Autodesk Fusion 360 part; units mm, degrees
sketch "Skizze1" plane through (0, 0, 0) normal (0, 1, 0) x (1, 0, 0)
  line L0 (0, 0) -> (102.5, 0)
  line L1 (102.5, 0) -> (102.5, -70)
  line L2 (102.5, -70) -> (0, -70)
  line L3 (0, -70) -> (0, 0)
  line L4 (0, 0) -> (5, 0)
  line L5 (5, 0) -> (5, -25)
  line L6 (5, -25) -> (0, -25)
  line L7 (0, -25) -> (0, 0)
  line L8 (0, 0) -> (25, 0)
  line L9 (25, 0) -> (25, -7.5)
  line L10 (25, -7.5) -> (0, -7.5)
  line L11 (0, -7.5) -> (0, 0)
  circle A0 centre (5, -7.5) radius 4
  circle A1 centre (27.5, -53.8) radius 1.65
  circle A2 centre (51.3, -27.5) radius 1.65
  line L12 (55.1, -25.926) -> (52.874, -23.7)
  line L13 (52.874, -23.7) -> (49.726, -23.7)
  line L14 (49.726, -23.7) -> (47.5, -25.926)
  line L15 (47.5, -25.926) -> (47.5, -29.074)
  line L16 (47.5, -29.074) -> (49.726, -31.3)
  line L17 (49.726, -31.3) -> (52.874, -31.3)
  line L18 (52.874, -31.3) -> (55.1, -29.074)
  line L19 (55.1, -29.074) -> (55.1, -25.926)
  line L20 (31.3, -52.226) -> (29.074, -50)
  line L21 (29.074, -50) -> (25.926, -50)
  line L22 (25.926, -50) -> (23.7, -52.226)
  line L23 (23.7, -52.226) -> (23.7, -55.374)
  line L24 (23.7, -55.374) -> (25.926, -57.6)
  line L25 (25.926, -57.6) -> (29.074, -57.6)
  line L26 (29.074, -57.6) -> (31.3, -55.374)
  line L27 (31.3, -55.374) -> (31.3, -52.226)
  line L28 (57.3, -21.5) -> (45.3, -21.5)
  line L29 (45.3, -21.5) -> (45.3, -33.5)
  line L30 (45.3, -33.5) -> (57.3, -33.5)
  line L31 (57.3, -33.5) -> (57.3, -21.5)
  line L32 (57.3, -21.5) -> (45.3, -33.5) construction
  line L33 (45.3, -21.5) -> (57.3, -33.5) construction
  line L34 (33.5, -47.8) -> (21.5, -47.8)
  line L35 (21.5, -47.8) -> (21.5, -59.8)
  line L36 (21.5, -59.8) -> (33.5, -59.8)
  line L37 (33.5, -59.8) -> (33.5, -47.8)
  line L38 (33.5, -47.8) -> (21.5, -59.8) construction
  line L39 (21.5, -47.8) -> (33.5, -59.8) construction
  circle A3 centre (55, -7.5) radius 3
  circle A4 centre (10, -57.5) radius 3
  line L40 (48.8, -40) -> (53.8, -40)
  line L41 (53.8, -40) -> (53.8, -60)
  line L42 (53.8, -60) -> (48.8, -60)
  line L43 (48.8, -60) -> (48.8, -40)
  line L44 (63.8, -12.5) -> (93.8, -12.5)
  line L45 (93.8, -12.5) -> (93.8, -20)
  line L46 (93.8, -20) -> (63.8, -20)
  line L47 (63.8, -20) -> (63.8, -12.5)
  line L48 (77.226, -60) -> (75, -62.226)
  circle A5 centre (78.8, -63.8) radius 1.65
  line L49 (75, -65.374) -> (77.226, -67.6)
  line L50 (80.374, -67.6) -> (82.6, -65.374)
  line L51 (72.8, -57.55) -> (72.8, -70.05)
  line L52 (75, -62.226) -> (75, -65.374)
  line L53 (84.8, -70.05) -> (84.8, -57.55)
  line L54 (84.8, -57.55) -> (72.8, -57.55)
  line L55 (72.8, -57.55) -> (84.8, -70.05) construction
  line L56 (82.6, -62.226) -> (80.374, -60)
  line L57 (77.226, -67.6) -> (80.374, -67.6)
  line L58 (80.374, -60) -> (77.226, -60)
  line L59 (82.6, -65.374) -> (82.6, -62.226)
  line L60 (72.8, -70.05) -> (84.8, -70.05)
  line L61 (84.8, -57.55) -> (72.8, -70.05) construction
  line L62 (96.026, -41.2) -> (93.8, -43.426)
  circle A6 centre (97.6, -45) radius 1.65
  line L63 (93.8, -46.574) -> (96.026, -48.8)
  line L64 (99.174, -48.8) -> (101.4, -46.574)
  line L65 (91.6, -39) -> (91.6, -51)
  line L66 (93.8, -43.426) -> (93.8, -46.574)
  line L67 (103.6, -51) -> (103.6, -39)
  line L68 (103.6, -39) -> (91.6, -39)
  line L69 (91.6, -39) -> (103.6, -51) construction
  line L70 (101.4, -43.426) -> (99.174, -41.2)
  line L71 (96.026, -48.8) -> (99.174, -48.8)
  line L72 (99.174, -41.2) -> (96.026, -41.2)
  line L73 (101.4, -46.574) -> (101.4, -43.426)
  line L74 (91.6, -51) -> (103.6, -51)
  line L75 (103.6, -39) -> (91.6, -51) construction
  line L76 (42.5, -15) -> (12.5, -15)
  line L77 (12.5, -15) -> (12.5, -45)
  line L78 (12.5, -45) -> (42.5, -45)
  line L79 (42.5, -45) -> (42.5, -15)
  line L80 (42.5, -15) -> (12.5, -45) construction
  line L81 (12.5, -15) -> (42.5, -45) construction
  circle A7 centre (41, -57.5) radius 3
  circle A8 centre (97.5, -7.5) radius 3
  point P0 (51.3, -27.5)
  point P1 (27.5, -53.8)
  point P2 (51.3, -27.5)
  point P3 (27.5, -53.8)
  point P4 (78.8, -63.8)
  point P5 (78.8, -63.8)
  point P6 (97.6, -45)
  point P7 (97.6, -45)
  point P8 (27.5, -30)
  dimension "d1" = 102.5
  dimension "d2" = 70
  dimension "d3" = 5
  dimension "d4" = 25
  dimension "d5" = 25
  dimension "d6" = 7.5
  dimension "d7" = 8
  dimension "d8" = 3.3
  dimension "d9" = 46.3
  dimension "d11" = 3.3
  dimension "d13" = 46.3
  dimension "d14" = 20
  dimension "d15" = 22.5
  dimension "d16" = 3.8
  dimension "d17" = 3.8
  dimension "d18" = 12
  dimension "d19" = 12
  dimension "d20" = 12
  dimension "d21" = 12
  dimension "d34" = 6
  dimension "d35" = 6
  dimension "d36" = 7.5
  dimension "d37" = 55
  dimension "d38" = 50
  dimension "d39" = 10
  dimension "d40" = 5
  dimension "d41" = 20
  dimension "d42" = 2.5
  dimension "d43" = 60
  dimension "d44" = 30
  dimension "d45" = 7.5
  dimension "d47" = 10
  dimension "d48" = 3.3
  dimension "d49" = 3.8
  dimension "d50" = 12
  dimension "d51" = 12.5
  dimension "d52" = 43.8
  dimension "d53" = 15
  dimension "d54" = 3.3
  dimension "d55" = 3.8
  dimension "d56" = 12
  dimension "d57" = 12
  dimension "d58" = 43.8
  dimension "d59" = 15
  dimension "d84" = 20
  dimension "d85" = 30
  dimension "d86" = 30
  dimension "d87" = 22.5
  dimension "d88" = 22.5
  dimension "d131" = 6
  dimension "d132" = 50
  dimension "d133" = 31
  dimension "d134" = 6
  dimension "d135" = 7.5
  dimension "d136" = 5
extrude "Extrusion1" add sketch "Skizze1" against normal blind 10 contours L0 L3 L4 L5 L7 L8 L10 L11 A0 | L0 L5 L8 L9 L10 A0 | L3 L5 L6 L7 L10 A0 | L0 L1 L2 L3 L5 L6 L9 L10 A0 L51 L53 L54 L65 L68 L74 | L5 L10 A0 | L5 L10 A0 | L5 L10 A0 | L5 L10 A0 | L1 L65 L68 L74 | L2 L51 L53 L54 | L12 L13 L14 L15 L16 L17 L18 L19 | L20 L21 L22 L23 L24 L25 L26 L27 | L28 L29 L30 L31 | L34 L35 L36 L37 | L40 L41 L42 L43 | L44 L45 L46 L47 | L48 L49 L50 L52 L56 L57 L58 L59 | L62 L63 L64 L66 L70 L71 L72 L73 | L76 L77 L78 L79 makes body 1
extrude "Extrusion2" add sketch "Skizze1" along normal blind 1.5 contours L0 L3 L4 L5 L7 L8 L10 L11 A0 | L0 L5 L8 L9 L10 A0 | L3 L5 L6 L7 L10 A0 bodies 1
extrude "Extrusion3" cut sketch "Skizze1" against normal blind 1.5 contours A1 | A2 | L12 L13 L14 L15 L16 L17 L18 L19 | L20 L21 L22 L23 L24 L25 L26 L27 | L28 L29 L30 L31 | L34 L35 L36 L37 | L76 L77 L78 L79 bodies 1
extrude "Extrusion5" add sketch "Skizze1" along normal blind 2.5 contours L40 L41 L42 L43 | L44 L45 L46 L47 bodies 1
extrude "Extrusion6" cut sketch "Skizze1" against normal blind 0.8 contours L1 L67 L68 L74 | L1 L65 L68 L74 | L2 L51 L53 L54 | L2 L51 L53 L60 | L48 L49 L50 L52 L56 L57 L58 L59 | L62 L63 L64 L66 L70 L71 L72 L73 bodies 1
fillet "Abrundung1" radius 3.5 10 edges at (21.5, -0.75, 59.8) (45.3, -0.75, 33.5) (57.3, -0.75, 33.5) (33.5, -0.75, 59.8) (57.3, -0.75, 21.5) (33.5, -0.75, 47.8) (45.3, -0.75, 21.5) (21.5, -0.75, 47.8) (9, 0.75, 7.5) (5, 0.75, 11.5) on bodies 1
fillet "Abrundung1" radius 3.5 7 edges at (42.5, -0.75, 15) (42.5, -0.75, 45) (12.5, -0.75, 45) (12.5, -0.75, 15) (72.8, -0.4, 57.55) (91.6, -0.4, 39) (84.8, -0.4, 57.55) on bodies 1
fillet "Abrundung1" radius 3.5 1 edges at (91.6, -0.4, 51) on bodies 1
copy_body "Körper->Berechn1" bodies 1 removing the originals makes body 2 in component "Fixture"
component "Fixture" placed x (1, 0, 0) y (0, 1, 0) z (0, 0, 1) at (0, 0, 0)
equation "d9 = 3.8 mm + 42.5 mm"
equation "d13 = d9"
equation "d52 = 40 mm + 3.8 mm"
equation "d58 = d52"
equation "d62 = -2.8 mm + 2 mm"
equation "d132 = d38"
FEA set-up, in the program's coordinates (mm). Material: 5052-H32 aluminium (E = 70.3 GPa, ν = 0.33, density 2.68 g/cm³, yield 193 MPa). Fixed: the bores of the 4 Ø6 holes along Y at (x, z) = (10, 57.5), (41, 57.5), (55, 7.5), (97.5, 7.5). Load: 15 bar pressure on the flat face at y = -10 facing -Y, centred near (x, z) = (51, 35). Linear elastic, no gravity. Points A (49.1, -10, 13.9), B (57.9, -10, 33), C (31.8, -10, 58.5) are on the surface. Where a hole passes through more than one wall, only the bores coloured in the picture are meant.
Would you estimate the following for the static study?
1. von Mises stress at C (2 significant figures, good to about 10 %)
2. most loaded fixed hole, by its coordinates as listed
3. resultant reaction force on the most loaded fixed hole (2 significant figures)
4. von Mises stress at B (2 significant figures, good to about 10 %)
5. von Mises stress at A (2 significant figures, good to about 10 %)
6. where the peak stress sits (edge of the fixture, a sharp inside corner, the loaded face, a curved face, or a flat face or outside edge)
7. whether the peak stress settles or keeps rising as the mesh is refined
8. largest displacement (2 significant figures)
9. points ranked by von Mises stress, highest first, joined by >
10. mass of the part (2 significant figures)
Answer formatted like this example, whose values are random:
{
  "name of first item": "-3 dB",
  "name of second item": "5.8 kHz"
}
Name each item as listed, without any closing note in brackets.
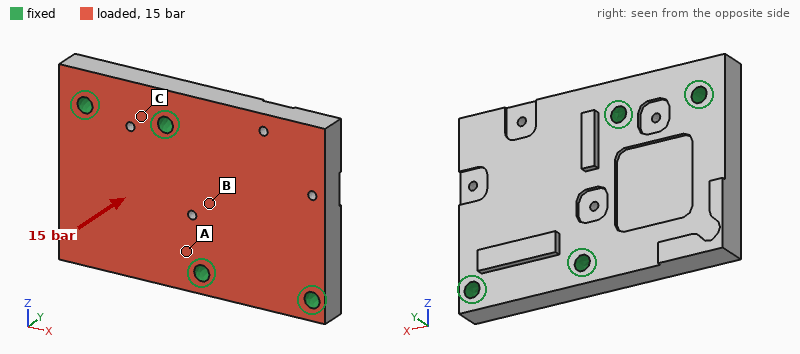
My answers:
{
  "von Mises stress at C": "13 MPa",
  "most loaded fixed hole, by its coordinates as listed": "(41, 57.5)",
  "resultant reaction force on the most loaded fixed hole": "3.6 kN",
  "von Mises stress at B": "29 MPa",
  "von Mises stress at A": "42 MPa",
  "where the peak stress sits": "edge of the fixture",
  "whether the peak stress settles or keeps rising as the mesh is refined": "keeps rising",
  "largest displacement": "0.18 mm",
  "points ranked by von Mises stress, highest first, joined by >": "A > B > C",
  "mass of the part": "190 g"
}
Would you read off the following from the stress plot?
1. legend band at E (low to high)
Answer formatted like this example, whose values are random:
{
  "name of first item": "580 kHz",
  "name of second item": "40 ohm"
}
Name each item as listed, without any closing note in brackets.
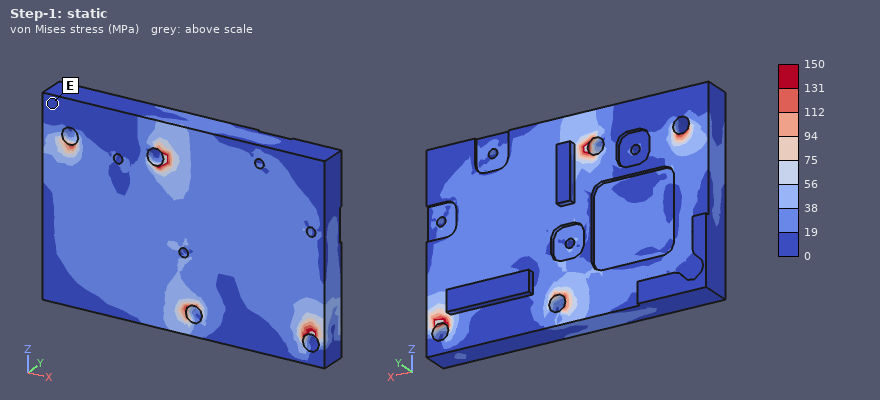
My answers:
{
  "legend band at E": "0 to 19 MPa"
}
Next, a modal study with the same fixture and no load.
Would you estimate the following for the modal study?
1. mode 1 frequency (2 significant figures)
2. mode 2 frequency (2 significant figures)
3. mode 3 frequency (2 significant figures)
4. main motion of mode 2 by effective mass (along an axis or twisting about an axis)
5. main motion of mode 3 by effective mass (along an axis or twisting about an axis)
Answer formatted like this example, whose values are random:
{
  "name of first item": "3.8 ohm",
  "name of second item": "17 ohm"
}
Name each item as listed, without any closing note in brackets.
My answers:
{
  "mode 1 frequency": "4000 Hz",
  "mode 2 frequency": "4600 Hz",
  "mode 3 frequency": "12 kHz",
  "main motion of mode 2 by effective mass": "along Y",
  "main motion of mode 3 by effective mass": "along Y"
}
